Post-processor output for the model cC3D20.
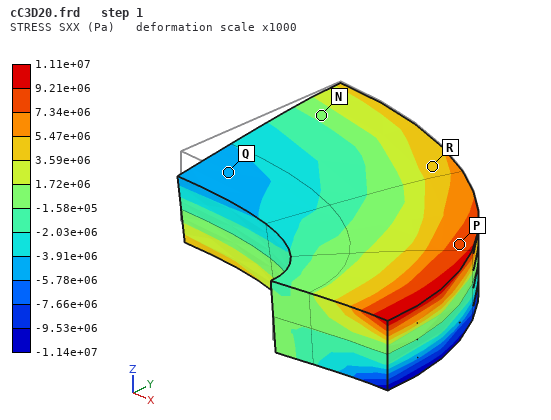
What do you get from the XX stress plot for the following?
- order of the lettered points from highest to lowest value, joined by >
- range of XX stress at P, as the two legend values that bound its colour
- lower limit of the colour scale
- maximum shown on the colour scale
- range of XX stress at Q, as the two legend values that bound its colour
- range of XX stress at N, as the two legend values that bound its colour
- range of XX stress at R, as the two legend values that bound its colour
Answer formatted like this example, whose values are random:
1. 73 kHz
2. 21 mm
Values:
1. P > R > N > Q
2. 7.34e+06 to 9.21e+06 Pa
3. -1.14e+07 Pa
4. 1.11e+07 Pa
5. -5.78e+06 to -3.91e+06 Pa
6. -1.58e+05 to 1.72e+06 Pa
7. 3.59e+06 to 5.47e+06 Pa
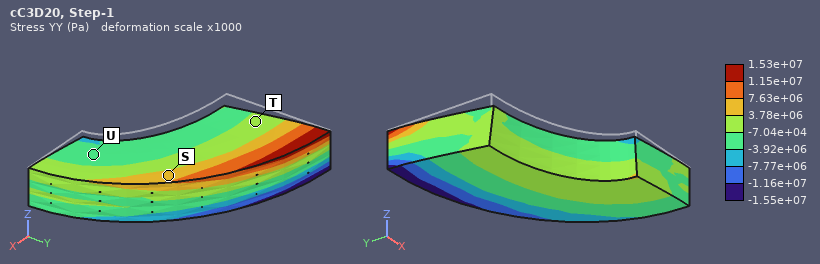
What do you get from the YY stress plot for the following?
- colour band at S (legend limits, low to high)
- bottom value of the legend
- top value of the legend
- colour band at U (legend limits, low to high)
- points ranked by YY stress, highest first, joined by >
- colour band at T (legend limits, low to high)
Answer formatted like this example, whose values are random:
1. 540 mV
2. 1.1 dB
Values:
1. 3.78e+06 to 7.63e+06 Pa
2. -1.55e+07 Pa
3. 1.53e+07 Pa
4. -3.92e+06 to -7.04e+04 Pa
5. S > T > U
6. -7.04e+04 to 3.78e+06 Pa
